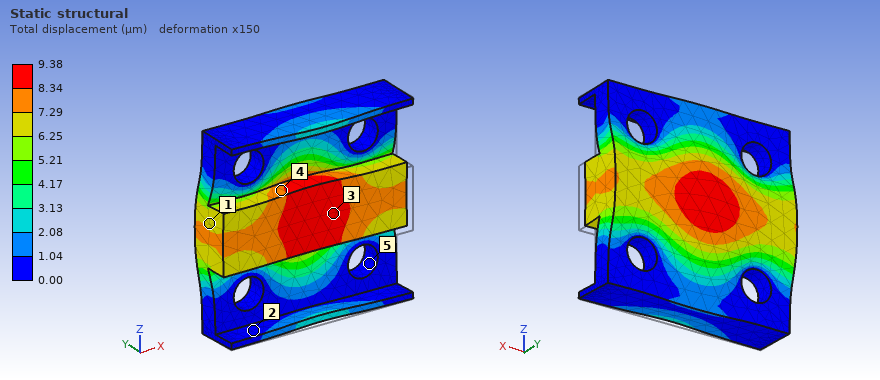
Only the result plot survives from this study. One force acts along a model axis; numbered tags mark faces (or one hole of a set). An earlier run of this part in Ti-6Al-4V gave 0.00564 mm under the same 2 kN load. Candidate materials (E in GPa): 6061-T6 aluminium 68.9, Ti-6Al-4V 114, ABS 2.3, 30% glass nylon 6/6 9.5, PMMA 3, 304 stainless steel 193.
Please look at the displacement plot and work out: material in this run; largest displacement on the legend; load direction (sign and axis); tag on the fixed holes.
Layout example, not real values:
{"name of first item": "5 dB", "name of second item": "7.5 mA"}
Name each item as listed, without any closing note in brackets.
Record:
{"material in this run": "6061-T6 aluminium", "largest displacement on the legend": "9.38 µm", "load direction": "+Y", "tag on the fixed holes": "5"}
